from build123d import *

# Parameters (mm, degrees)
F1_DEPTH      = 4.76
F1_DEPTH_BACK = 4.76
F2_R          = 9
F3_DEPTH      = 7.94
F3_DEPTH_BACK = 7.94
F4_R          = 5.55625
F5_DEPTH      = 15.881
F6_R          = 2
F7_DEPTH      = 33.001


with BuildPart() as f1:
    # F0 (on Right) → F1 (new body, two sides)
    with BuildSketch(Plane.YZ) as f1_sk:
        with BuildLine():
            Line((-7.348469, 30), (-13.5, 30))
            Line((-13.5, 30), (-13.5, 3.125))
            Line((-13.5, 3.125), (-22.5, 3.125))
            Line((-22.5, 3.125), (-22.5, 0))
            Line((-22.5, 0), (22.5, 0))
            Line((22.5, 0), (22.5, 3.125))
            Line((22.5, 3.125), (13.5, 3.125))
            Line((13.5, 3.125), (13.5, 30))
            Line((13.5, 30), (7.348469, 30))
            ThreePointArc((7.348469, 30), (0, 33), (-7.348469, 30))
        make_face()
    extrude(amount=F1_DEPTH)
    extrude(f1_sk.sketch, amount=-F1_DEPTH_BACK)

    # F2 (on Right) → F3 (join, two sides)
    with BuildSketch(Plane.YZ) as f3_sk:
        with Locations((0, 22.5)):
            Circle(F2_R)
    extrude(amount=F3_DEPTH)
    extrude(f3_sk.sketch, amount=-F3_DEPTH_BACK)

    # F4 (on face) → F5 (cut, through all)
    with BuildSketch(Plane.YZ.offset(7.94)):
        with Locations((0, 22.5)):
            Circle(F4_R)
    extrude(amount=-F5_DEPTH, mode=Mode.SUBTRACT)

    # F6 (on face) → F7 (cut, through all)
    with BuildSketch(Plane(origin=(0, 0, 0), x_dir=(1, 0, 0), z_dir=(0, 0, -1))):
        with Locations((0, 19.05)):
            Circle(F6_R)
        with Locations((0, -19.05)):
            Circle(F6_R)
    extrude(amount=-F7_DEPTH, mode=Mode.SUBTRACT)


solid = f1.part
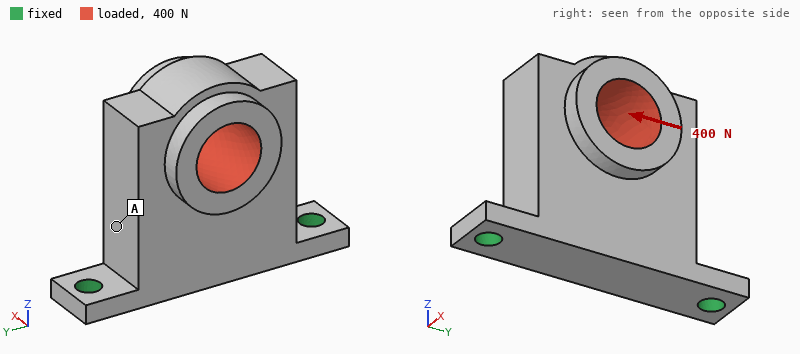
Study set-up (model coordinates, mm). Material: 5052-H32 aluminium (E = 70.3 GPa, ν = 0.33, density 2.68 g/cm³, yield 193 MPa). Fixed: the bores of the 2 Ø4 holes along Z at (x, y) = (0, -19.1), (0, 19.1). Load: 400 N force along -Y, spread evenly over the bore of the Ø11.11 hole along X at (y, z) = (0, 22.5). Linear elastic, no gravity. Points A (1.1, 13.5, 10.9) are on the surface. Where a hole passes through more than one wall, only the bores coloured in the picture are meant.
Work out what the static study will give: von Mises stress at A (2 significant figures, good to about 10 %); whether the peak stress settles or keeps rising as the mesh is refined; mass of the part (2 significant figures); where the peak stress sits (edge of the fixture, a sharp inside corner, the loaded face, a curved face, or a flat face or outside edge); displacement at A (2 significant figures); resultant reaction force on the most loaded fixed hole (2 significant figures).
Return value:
5.3 MPa
keeps rising
23 g
edge of the fixture
6.5 µm
340 N
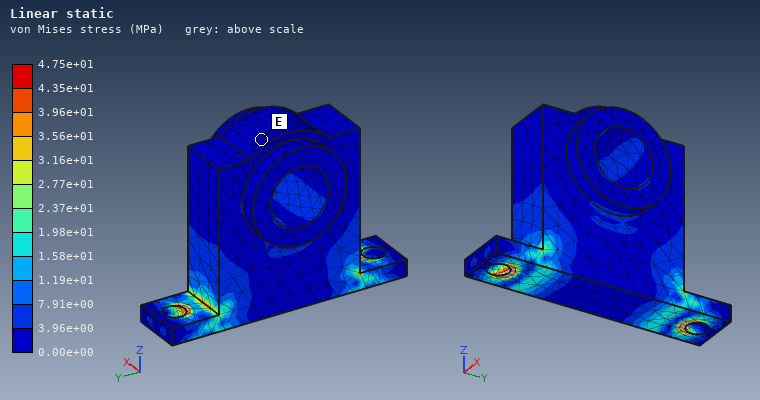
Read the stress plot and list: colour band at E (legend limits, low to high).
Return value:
0.00e+00 to 3.96e+00 MPa
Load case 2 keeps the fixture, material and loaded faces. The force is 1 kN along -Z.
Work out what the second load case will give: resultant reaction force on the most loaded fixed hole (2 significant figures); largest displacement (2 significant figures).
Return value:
560 N
12 µm
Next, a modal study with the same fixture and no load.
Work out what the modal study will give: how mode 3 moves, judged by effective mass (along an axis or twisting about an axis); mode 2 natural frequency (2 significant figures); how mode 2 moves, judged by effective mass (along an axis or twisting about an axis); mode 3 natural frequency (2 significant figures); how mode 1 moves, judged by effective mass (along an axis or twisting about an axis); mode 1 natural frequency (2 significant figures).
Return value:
along Z
8100 Hz
along Y
10 kHz
along X
2000 Hz
